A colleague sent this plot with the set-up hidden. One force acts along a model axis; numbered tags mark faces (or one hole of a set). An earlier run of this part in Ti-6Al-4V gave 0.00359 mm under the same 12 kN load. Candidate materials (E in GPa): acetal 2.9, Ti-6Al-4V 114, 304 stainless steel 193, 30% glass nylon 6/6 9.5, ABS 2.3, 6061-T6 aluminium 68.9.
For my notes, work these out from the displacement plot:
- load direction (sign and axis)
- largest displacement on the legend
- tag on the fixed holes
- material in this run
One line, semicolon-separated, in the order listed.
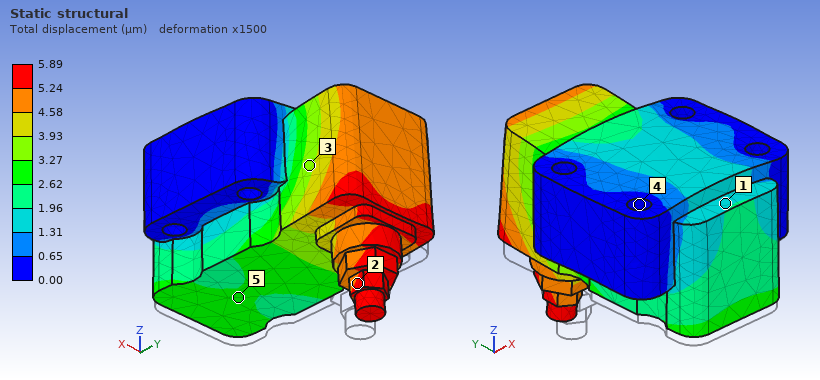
+Z; 5.89 µm; 4; 6061-T6 aluminium
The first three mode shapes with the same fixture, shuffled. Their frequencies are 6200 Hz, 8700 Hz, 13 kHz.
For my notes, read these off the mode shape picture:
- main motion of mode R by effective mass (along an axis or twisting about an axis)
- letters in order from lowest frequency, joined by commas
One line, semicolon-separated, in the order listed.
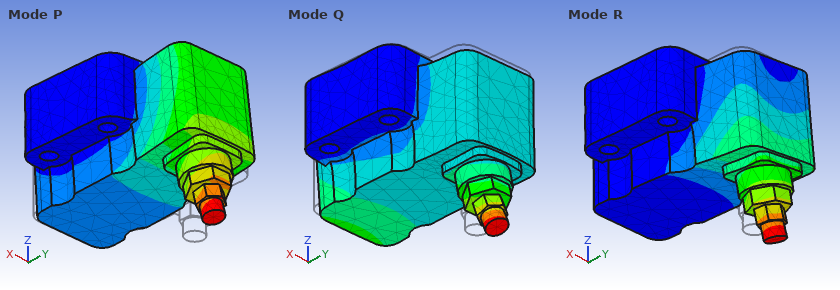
along X; P, R, Q
